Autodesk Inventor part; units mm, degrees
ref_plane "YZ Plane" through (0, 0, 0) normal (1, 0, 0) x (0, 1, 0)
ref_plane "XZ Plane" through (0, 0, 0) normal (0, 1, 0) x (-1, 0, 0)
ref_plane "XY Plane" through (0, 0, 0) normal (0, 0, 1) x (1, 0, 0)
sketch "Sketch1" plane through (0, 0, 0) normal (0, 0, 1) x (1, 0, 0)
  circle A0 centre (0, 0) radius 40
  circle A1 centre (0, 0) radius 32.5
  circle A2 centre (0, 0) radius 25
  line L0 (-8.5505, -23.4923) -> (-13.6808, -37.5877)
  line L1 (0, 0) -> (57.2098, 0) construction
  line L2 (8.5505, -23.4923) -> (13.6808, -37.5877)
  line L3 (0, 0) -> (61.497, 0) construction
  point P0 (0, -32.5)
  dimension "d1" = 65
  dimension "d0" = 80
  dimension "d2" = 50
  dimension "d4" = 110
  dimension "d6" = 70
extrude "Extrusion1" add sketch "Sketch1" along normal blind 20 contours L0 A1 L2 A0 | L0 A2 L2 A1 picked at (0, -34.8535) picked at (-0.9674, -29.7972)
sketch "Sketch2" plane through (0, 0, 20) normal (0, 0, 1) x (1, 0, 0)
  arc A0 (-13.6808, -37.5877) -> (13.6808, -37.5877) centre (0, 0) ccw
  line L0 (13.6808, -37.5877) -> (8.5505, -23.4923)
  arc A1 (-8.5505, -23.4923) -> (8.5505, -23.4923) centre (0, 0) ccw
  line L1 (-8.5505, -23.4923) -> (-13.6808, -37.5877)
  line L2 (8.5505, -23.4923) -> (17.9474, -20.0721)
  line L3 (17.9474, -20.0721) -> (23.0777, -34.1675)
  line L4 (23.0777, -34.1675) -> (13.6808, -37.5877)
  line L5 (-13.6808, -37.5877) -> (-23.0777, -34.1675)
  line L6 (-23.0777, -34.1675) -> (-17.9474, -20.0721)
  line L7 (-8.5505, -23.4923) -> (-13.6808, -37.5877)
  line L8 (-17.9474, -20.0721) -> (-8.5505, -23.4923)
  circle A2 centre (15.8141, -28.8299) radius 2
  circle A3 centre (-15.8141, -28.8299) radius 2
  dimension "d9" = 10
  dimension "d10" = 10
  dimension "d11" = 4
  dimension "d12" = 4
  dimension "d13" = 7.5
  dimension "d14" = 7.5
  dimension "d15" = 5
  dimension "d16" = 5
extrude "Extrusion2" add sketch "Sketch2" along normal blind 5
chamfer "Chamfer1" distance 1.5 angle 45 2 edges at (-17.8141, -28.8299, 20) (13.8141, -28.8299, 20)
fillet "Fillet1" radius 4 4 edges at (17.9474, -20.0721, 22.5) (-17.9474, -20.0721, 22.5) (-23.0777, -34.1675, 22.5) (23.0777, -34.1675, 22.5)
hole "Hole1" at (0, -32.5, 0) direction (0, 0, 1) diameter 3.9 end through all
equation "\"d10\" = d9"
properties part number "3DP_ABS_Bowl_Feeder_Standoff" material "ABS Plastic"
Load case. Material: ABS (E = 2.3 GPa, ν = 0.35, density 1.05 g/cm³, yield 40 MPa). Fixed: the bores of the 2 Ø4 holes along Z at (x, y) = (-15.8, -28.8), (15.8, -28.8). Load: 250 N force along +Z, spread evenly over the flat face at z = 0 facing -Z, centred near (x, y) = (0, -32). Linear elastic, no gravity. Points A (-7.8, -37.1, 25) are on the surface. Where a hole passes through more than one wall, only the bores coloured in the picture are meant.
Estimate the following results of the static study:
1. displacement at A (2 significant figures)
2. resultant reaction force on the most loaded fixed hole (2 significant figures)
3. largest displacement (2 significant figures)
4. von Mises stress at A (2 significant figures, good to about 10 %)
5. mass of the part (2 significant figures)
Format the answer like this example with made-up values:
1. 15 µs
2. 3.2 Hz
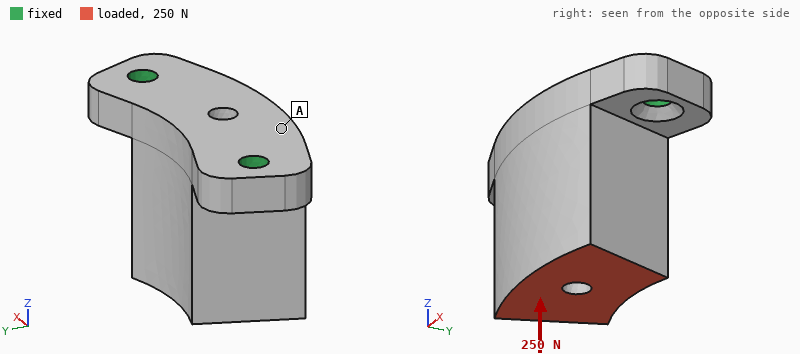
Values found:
1. 0.073 mm
2. 140 N
3. 0.16 mm
4. 2.3 MPa
5. 10.0 g
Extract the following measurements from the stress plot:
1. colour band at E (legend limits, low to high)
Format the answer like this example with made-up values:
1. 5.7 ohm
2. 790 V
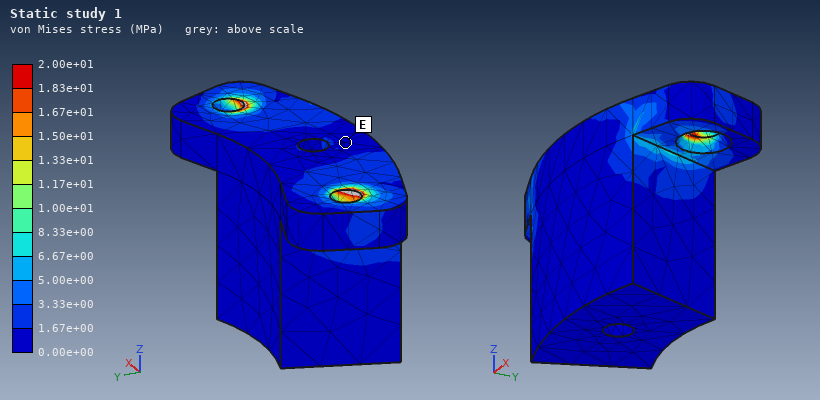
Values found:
1. 0.00e+00 to 1.67e+00 MPa
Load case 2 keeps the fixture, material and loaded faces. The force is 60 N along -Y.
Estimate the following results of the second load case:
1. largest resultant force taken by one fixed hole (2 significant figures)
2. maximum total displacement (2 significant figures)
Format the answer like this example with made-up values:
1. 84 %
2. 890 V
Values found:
1. 35 N
2. 0.31 mm
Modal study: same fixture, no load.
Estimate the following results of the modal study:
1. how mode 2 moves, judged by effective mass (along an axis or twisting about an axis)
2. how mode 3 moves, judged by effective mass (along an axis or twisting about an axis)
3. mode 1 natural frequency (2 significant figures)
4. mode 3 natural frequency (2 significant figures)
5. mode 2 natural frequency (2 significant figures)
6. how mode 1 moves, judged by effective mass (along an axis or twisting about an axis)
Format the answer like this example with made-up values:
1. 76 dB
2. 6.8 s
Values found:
1. along X
2. along Z
3. 1300 Hz
4. 4600 Hz
5. 4100 Hz
6. along Y
